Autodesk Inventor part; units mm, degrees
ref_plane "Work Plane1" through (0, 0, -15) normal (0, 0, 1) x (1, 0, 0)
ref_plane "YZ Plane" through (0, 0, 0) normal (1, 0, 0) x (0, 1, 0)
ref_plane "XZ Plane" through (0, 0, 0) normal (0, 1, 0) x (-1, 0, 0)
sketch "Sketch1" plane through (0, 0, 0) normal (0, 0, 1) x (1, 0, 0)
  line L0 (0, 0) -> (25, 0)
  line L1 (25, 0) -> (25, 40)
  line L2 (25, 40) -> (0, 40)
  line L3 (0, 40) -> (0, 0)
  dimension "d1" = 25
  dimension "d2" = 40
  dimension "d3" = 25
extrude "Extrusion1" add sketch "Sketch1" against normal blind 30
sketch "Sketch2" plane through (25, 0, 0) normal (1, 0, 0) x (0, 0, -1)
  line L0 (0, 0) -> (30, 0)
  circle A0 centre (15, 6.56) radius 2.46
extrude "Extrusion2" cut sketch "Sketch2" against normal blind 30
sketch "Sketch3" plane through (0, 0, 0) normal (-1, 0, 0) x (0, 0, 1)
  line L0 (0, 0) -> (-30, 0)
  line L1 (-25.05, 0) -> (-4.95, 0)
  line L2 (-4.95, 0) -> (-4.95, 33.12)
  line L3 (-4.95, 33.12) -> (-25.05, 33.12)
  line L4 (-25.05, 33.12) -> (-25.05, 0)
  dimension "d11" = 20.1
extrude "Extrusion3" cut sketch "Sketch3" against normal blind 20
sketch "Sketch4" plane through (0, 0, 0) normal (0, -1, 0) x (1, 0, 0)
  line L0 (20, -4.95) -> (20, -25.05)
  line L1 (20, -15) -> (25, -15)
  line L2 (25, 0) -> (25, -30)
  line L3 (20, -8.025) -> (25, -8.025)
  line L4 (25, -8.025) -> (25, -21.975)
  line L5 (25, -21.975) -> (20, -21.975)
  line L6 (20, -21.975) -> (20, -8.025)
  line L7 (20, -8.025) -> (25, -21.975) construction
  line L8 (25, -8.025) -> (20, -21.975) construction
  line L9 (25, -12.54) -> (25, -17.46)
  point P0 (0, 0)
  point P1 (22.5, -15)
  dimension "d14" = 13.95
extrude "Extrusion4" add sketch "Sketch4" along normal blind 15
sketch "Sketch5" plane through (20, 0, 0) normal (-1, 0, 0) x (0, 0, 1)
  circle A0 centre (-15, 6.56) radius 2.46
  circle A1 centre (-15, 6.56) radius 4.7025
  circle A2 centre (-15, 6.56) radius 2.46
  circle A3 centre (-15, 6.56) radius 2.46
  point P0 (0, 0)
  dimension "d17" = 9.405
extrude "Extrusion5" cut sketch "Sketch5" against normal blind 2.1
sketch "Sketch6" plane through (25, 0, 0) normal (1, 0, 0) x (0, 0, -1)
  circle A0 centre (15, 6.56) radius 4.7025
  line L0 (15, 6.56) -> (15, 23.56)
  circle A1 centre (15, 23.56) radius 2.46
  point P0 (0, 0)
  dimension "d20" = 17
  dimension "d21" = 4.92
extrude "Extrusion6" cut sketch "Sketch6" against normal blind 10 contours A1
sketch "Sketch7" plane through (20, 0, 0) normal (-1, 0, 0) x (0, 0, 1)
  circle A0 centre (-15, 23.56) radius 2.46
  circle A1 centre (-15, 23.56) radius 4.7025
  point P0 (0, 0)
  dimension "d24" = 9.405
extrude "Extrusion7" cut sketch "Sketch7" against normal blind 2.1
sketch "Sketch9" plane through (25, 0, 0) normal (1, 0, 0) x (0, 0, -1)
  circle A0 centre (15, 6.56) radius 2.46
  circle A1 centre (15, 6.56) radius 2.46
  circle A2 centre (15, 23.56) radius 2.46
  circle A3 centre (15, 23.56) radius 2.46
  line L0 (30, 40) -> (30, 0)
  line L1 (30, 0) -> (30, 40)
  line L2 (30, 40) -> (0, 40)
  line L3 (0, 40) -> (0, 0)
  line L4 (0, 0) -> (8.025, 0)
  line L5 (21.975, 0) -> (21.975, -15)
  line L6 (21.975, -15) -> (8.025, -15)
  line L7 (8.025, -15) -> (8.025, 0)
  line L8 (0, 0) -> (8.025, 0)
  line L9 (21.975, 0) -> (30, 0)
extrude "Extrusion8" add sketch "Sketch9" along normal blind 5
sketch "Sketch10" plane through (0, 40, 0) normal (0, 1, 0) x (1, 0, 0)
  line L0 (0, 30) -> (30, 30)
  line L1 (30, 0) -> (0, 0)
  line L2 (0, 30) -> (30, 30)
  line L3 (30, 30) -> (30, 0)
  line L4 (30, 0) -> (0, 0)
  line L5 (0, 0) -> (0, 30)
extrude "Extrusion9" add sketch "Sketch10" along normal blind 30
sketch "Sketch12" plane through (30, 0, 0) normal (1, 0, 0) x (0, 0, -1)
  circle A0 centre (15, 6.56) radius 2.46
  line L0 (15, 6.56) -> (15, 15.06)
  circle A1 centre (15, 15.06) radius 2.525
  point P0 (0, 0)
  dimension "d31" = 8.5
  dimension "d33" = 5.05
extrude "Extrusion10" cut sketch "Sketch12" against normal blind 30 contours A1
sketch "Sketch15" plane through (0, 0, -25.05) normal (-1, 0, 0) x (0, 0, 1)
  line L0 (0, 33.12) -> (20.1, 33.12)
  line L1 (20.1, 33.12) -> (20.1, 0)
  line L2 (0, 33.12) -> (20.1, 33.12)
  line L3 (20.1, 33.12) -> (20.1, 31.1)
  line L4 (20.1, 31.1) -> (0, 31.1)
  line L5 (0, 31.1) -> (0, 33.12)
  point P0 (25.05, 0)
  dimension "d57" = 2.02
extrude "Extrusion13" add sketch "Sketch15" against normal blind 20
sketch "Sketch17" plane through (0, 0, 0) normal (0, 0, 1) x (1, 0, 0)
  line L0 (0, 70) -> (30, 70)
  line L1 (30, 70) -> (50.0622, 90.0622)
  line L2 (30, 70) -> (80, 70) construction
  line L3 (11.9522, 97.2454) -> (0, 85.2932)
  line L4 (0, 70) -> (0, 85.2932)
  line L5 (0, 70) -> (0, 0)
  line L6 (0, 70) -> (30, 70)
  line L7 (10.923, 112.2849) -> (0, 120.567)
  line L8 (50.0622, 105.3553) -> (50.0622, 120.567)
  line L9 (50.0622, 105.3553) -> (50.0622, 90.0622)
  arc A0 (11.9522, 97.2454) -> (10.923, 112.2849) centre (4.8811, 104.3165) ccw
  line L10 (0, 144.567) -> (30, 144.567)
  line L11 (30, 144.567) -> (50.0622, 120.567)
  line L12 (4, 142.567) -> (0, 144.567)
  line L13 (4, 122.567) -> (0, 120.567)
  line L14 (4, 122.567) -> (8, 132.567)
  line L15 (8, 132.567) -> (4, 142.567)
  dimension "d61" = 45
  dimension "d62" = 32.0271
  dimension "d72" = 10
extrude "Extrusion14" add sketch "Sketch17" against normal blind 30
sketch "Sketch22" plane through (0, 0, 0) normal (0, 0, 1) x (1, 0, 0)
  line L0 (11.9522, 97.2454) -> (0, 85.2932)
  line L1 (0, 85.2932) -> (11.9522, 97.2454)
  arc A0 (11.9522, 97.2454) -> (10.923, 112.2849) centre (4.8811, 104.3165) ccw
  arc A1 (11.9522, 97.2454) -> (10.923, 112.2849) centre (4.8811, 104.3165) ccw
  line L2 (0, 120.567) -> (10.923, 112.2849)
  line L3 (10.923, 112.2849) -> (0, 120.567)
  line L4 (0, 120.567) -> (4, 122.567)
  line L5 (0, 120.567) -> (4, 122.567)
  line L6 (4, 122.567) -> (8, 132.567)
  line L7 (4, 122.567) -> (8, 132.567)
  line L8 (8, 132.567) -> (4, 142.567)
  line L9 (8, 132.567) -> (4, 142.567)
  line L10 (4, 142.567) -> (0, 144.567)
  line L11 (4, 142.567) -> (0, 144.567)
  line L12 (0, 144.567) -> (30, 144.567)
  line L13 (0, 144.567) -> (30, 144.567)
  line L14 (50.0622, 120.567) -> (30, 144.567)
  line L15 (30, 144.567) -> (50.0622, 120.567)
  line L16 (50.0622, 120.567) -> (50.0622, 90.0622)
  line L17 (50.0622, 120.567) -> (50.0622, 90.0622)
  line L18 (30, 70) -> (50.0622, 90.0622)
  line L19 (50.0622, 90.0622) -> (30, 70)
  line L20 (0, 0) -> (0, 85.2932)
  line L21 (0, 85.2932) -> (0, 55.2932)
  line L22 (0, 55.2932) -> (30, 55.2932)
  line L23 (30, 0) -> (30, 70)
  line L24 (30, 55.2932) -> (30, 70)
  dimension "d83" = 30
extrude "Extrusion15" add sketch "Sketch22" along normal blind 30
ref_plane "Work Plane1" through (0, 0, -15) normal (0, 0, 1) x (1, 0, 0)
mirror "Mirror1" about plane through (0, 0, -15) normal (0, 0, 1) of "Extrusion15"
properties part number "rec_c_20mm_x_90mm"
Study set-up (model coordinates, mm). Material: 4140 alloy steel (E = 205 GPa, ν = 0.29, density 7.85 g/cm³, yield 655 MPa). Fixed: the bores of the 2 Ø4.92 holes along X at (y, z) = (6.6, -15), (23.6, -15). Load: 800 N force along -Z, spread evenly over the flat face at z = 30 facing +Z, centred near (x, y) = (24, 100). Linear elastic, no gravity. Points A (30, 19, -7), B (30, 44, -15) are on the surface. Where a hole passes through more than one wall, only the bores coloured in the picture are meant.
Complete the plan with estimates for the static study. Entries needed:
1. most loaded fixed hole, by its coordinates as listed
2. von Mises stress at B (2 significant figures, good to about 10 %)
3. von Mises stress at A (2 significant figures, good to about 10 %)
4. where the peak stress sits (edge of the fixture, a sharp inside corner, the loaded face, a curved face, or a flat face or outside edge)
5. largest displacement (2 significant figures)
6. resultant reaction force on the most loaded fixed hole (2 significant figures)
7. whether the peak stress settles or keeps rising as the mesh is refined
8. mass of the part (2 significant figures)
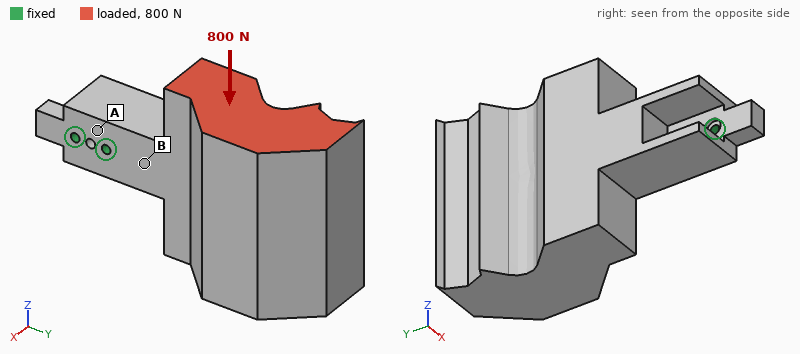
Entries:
(23.6, -15)
7.7 MPa
20 MPa
edge of the fixture
54 µm
3.4 kN
keeps rising
2.6 kg
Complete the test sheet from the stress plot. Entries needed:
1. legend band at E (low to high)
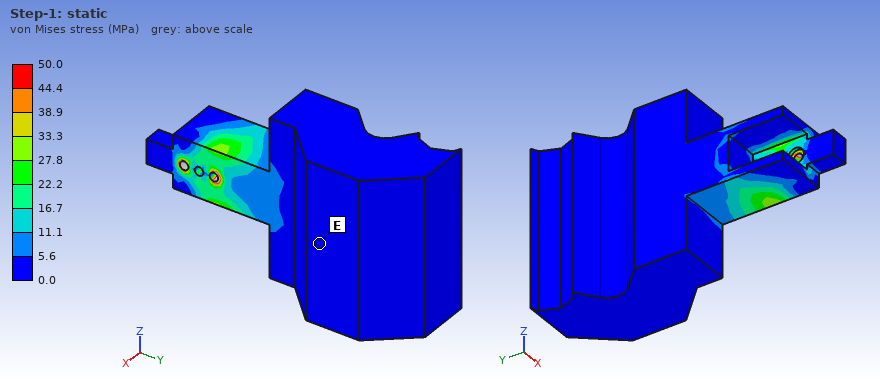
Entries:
0.0 to 5.6 MPa
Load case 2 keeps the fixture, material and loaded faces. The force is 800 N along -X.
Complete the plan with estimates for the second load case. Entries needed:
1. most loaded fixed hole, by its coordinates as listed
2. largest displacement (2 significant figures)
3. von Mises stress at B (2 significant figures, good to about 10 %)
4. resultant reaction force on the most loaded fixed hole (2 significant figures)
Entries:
(23.6, -15)
0.10 mm
18 MPa
3.2 kN
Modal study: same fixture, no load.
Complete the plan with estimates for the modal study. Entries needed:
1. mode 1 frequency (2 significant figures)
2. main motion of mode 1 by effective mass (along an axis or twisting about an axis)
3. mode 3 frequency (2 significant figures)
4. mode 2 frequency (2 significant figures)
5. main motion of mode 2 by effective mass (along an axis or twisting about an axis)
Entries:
430 Hz
along X
830 Hz
470 Hz
along Z
